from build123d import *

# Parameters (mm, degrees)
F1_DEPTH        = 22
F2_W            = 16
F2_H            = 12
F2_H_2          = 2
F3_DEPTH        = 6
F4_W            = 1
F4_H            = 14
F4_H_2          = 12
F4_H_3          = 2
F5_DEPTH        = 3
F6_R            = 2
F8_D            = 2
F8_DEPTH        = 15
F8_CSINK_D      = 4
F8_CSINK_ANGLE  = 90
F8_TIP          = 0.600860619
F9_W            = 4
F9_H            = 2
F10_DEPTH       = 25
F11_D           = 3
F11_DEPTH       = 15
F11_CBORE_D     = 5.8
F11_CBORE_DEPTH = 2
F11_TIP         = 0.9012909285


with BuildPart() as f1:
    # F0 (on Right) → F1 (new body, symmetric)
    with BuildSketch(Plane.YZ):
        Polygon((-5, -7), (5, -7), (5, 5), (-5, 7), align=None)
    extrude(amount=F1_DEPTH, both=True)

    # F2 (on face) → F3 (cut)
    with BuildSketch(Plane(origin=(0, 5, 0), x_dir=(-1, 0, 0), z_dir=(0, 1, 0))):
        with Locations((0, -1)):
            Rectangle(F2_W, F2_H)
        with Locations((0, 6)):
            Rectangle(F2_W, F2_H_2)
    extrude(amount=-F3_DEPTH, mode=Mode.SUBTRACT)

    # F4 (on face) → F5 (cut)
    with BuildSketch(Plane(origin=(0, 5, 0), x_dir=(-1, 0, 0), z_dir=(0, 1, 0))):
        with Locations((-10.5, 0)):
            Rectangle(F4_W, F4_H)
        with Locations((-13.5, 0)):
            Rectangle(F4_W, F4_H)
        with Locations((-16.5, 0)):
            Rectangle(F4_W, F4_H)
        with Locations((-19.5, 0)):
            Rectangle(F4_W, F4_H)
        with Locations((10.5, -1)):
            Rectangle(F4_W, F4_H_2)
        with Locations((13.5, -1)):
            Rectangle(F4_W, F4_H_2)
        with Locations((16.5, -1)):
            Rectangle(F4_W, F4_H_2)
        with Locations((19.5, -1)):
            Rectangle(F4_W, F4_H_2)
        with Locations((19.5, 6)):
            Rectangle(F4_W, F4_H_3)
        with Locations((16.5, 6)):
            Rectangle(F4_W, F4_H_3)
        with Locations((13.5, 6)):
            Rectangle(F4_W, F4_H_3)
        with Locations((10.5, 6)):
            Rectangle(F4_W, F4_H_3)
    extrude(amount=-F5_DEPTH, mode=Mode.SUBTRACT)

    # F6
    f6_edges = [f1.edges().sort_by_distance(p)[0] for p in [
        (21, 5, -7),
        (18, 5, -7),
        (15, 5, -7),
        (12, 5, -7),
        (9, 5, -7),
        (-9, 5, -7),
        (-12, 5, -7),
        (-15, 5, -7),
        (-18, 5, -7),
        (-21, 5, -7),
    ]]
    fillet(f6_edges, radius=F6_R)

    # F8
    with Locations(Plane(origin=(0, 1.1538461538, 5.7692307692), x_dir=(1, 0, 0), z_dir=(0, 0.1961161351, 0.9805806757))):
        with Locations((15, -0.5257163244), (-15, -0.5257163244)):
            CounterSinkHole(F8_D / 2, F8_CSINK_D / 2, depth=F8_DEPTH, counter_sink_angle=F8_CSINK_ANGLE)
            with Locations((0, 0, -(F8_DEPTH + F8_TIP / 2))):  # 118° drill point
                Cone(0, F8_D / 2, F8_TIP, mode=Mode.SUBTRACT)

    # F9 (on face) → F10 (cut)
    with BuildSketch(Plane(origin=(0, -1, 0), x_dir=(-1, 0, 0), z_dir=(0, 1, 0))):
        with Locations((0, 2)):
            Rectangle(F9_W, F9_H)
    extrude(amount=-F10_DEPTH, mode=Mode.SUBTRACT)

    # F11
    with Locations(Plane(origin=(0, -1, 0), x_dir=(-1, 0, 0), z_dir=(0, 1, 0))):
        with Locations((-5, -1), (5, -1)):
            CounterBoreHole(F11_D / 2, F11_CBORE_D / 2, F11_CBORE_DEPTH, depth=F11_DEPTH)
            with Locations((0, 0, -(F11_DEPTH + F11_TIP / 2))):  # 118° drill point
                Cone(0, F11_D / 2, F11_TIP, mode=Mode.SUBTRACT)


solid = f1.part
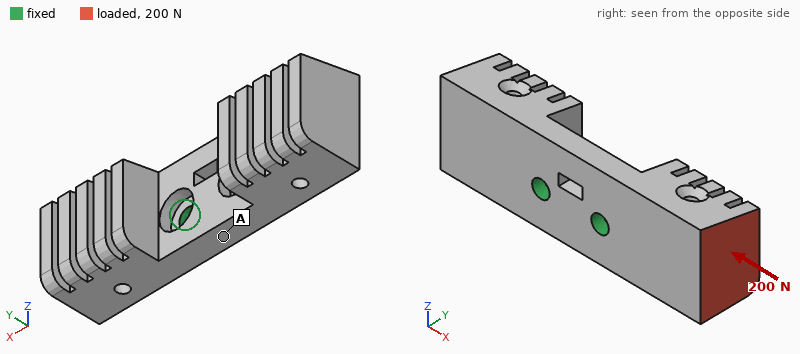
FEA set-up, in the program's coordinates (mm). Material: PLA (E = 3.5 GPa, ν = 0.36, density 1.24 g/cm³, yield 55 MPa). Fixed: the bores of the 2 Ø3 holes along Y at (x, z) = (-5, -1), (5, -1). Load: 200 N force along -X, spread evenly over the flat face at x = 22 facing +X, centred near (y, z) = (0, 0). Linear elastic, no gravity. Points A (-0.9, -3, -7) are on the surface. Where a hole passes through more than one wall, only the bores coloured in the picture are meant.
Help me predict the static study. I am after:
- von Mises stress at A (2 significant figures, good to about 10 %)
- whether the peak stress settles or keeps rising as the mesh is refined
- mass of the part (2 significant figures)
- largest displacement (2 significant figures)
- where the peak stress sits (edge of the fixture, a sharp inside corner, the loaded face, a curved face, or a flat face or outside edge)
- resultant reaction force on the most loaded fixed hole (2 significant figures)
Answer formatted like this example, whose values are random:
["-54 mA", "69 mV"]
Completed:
["5.5 MPa", "keeps rising", "4.9 g", "0.42 mm", "edge of the fixture", "120 N"]
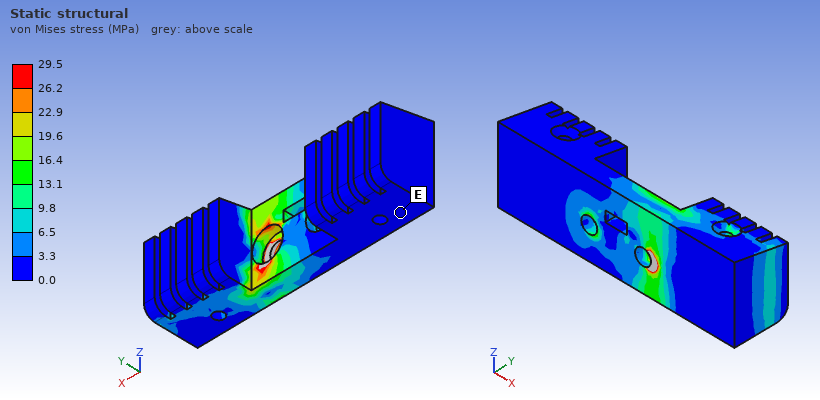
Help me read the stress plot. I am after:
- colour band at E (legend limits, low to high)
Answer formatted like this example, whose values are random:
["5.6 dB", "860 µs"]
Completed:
["0.0 to 3.3 MPa"]
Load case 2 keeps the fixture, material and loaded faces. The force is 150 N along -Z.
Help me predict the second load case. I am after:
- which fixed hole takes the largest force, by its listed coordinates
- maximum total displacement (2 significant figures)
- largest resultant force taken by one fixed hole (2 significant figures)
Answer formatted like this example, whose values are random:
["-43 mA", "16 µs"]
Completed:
["(5, -1)", "0.40 mm", "310 N"]
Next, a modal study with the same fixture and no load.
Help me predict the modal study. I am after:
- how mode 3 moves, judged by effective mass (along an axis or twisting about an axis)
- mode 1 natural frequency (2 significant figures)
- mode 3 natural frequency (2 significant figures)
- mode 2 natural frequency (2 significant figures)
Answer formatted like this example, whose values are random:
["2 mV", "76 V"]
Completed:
["along Z", "1900 Hz", "3100 Hz", "1900 Hz"]
